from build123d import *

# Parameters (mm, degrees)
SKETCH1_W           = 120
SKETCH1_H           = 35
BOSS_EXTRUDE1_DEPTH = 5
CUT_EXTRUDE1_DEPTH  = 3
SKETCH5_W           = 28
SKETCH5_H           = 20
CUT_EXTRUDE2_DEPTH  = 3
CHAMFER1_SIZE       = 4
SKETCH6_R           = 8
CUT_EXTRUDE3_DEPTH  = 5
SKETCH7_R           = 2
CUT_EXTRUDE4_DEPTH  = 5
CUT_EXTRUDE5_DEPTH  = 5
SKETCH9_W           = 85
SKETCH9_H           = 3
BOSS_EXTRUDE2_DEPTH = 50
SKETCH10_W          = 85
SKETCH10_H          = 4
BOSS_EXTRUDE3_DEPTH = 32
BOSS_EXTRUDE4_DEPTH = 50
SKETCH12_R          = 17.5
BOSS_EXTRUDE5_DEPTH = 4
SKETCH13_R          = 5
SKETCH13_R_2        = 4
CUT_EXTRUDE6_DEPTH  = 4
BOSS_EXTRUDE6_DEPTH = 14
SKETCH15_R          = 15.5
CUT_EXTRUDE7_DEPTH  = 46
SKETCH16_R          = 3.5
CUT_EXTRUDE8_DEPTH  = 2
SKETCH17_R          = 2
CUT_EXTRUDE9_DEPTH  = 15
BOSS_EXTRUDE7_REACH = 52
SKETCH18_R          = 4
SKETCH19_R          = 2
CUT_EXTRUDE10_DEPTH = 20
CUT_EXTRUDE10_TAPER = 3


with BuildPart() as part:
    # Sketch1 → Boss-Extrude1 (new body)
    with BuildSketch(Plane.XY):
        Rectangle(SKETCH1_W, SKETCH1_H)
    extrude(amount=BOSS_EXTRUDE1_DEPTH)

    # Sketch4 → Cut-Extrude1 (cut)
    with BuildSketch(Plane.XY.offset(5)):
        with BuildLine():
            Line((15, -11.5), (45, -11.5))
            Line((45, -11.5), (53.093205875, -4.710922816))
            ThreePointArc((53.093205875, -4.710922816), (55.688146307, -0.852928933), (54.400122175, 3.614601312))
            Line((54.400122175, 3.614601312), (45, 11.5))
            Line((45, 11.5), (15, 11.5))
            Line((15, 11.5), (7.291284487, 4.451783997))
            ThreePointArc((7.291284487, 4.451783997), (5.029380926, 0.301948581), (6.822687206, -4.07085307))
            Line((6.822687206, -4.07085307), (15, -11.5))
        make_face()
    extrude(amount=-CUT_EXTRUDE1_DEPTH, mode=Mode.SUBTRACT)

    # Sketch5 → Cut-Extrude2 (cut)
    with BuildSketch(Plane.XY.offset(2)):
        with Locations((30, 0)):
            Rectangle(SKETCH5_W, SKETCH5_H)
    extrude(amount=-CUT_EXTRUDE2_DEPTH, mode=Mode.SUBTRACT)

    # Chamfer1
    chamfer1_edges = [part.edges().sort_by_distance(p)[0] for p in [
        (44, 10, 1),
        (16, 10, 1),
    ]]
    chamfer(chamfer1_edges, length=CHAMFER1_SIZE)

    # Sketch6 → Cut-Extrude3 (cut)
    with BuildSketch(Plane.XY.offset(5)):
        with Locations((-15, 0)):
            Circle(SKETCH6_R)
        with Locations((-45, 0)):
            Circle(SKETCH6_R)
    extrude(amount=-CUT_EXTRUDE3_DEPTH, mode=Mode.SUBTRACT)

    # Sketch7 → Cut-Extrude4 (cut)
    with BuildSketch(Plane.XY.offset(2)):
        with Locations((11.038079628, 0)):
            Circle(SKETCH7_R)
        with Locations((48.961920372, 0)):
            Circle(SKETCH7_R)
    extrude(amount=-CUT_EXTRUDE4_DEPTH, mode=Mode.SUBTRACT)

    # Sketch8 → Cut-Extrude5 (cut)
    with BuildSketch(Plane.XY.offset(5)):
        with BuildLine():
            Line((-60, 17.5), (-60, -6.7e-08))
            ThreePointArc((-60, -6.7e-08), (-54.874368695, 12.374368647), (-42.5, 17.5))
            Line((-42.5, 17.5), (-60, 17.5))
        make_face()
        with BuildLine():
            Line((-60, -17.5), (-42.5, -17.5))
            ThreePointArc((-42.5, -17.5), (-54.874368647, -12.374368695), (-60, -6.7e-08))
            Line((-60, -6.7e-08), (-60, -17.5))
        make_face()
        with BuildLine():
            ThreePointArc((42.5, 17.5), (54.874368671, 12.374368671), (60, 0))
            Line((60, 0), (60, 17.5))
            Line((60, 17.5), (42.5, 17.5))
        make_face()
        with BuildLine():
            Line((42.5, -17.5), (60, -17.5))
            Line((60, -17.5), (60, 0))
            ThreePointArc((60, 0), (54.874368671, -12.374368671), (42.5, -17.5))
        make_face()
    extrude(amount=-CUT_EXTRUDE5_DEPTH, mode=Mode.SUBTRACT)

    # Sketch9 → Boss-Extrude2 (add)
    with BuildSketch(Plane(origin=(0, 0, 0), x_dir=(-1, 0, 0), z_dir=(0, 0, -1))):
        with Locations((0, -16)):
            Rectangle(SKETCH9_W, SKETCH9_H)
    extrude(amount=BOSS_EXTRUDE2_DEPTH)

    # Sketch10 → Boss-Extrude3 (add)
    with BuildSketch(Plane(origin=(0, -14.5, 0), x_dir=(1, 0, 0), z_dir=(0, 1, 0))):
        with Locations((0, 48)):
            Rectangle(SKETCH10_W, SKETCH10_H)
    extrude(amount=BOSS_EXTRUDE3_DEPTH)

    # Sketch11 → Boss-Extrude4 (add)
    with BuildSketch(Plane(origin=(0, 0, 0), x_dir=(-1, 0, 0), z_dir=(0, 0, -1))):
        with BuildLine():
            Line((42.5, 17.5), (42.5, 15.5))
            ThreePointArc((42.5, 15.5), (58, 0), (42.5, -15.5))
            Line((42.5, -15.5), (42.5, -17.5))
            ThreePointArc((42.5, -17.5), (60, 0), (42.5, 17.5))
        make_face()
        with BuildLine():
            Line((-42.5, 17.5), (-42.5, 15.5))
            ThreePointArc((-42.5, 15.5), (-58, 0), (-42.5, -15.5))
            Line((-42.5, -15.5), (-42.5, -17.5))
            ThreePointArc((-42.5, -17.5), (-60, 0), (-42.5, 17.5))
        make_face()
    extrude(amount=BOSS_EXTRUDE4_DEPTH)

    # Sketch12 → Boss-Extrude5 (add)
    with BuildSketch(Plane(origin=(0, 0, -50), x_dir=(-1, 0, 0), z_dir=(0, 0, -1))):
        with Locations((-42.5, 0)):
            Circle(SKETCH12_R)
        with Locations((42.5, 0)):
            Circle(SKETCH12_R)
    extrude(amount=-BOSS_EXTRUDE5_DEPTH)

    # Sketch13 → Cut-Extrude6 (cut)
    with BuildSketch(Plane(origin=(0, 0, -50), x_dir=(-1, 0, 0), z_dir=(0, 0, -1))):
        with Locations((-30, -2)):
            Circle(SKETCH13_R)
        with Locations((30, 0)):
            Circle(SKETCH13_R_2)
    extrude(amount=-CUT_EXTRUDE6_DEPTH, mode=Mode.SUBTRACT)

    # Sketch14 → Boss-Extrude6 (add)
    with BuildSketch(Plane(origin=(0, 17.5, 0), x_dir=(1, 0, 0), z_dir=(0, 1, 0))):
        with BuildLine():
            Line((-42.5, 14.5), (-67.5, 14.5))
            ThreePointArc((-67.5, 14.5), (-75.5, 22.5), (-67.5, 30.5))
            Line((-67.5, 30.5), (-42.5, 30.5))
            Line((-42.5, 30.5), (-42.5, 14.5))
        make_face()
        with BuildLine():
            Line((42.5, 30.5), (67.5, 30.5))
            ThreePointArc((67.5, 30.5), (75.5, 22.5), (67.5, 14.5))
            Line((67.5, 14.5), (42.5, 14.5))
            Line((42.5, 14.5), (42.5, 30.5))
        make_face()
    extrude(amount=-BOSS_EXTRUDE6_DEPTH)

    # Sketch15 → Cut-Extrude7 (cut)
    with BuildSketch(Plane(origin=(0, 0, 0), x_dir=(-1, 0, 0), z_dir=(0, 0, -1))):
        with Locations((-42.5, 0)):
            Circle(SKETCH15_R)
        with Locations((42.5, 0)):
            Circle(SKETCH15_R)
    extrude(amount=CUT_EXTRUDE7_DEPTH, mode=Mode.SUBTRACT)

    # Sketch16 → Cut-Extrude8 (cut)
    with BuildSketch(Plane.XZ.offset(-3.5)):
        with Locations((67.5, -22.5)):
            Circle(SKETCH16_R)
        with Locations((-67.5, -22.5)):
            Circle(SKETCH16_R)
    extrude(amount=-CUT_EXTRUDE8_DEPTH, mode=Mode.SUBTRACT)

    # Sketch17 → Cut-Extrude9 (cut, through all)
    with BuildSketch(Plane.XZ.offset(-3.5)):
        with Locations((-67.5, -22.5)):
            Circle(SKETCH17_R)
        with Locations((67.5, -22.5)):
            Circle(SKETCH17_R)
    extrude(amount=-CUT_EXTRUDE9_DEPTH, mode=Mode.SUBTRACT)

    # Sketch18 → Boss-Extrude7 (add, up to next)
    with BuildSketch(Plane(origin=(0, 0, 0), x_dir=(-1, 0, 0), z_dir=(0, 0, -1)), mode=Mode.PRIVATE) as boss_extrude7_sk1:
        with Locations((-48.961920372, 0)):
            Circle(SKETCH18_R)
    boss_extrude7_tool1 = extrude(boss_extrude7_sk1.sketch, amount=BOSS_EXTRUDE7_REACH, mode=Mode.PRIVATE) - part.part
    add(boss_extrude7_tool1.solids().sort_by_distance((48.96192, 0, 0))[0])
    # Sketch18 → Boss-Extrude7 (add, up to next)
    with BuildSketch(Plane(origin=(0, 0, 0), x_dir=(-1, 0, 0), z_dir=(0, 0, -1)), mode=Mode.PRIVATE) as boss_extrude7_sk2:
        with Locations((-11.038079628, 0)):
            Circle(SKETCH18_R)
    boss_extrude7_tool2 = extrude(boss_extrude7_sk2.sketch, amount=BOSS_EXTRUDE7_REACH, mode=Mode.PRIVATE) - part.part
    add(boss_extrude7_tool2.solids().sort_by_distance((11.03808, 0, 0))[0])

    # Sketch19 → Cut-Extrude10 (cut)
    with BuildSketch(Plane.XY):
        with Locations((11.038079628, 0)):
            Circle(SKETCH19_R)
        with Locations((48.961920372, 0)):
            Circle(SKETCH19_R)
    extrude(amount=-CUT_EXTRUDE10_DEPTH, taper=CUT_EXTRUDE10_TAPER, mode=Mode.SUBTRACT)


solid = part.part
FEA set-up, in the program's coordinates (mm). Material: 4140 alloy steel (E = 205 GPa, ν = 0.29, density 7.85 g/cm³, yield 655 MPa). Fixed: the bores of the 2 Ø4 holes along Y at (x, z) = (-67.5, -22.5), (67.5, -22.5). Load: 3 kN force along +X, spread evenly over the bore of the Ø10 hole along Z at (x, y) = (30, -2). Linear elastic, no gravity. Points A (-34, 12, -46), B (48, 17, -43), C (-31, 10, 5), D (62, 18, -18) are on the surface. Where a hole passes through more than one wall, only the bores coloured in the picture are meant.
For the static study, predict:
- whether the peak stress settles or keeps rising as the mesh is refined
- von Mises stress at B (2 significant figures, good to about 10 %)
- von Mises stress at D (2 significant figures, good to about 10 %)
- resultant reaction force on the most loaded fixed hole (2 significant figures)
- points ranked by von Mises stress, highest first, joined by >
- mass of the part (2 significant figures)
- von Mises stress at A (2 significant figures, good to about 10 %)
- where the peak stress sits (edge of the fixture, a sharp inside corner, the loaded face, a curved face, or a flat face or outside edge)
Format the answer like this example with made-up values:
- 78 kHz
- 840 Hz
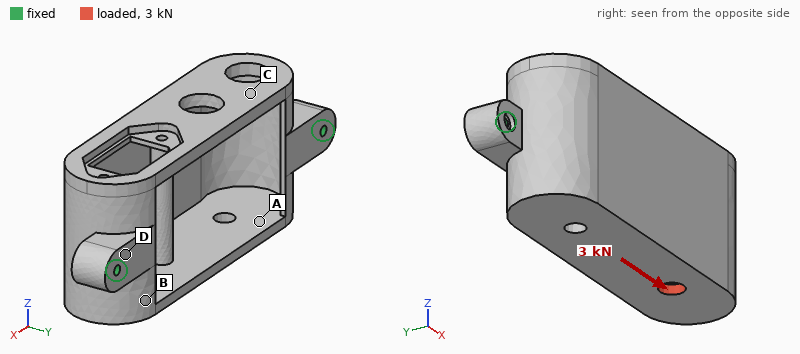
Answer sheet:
- keeps rising
- 55 MPa
- 21 MPa
- 1.6 kN
- B > A > D > C
- 490 g
- 31 MPa
- edge of the fixture
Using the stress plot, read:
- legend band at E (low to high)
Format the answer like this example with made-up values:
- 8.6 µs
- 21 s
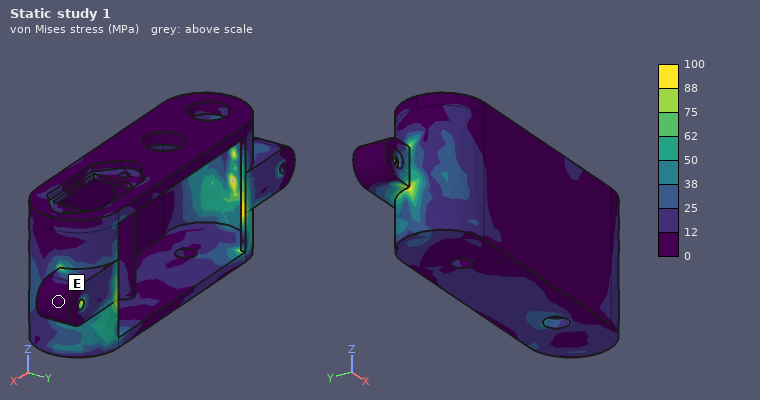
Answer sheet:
- 0 to 12 MPa
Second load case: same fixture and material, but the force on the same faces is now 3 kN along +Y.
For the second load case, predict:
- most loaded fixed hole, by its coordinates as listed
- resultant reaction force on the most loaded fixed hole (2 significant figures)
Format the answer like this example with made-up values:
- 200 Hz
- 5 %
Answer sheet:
- (67.5, -22.5)
- 2.3 kN
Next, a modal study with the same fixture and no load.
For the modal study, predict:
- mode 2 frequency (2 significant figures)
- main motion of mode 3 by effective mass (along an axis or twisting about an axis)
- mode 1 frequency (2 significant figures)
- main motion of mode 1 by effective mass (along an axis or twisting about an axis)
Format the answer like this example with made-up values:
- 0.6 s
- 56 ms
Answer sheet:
- 2900 Hz
- along X
- 2000 Hz
- along Z
